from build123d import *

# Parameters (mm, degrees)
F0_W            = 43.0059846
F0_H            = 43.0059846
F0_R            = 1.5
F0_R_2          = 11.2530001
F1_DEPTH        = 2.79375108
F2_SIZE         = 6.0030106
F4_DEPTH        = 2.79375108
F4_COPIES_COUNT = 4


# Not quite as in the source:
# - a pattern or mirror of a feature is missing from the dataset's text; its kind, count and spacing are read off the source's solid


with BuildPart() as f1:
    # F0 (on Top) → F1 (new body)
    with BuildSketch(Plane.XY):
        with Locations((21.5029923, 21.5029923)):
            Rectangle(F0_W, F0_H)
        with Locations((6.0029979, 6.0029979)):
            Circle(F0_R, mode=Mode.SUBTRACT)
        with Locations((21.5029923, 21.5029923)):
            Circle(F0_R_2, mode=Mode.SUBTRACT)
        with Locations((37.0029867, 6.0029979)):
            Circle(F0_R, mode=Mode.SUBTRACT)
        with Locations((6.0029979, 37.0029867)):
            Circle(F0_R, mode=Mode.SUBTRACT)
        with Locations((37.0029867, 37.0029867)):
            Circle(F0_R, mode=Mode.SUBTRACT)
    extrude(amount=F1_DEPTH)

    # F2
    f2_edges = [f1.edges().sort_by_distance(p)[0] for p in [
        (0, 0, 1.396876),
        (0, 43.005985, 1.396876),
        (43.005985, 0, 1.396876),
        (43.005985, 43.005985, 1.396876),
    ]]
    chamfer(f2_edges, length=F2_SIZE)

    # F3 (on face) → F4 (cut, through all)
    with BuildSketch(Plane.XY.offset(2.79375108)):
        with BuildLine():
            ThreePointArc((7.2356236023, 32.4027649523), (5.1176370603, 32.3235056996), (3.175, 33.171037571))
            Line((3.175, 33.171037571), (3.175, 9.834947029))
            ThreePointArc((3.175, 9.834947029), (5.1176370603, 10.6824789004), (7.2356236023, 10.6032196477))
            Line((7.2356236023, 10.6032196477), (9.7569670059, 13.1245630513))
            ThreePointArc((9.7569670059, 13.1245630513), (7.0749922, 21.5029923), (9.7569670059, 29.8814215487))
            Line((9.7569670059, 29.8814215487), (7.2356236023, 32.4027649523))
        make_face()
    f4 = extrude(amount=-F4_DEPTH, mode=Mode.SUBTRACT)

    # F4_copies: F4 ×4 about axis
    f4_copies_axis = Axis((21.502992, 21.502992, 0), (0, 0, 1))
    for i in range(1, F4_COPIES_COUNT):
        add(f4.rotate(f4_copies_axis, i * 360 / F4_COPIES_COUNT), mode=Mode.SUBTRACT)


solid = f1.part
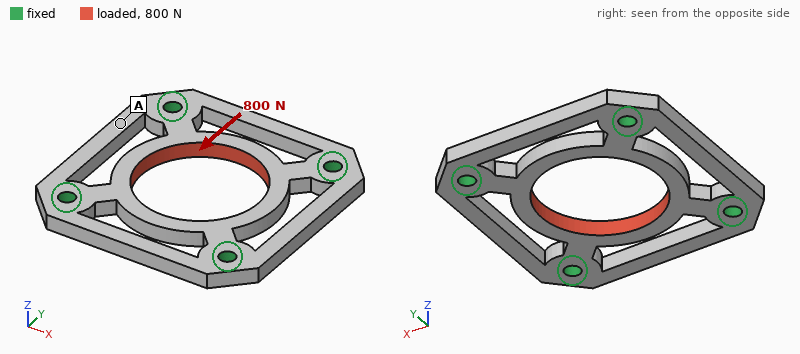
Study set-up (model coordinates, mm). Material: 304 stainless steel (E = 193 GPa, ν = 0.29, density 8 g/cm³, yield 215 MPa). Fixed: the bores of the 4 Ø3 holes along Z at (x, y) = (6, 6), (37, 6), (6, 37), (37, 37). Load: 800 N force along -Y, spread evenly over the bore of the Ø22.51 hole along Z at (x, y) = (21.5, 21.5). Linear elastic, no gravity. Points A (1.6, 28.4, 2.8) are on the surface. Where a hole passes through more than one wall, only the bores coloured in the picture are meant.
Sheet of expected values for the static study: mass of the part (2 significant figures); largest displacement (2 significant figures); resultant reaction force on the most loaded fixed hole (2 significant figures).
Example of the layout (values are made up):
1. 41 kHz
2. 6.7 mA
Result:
1. 21 g
2. 6.9 µm
3. 200 N
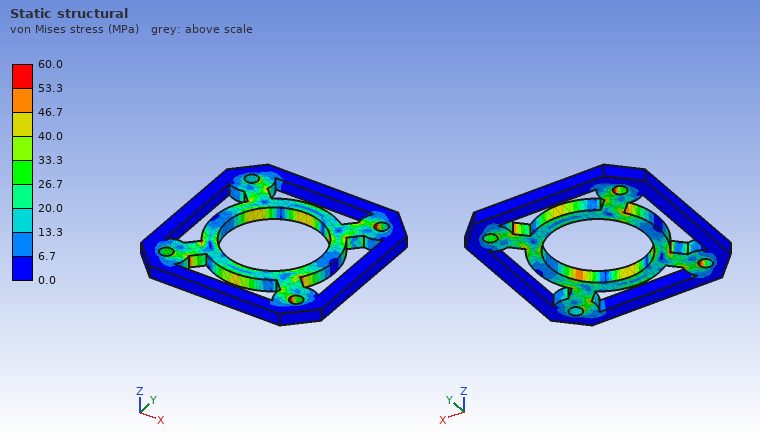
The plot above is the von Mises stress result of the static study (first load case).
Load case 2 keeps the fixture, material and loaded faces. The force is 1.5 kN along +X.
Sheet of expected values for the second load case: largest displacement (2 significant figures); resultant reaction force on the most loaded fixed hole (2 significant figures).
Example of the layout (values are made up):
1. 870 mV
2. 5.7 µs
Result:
1. 13 µm
2. 380 N
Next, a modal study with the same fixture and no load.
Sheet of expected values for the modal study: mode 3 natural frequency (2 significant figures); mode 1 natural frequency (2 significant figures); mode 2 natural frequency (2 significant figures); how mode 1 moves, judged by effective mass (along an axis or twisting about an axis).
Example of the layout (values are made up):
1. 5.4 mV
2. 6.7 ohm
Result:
1. 15 kHz
2. 14 kHz
3. 15 kHz
4. along Z
